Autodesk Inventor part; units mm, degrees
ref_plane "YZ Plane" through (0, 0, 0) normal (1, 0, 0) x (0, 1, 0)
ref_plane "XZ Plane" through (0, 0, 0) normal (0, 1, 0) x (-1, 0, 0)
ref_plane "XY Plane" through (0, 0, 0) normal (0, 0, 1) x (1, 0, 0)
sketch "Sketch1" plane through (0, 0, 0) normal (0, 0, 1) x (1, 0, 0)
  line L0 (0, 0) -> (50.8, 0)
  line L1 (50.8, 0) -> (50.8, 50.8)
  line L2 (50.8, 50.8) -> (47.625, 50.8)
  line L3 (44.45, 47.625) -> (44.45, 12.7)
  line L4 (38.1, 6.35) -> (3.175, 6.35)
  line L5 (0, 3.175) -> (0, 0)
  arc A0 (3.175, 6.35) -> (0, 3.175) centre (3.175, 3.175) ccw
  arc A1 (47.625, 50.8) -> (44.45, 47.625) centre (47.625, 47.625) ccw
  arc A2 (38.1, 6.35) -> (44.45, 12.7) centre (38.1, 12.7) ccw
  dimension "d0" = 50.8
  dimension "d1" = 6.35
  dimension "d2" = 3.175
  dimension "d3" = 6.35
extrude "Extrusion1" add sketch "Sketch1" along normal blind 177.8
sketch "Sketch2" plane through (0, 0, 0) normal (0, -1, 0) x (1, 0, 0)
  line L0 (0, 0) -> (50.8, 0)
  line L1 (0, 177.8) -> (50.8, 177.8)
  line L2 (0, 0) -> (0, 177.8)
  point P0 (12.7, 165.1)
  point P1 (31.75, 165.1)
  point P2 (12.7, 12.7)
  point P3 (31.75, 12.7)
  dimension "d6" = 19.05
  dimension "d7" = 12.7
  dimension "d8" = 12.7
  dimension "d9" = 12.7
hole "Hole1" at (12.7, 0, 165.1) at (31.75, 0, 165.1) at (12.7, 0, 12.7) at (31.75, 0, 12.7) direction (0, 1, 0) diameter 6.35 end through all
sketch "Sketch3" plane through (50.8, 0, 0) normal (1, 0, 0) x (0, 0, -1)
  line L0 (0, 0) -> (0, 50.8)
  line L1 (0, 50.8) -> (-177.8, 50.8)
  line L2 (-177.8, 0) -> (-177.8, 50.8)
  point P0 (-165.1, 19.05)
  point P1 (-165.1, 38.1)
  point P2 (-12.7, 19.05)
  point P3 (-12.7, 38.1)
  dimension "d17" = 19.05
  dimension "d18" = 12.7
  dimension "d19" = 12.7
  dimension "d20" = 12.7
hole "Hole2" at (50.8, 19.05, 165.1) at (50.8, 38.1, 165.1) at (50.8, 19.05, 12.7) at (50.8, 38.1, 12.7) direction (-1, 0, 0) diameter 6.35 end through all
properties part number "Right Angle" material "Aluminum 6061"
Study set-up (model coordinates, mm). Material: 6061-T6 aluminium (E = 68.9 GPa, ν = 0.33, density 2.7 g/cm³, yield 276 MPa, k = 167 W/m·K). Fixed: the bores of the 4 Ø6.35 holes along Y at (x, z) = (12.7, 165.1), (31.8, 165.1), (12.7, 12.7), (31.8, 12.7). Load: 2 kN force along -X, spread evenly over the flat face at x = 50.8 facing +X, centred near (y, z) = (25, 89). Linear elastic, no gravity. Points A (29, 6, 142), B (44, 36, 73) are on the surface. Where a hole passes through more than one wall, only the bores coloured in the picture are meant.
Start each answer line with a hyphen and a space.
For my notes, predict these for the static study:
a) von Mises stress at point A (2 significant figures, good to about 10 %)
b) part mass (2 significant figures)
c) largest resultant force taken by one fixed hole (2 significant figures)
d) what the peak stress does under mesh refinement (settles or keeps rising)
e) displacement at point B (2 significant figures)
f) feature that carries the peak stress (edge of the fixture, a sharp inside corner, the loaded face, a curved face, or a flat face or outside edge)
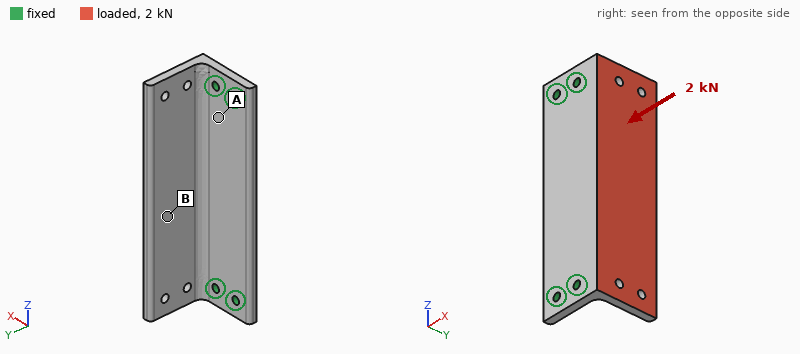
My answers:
- 30 MPa
- 290 g
- 1.0 kN
- keeps rising
- 0.18 mm
- edge of the fixture
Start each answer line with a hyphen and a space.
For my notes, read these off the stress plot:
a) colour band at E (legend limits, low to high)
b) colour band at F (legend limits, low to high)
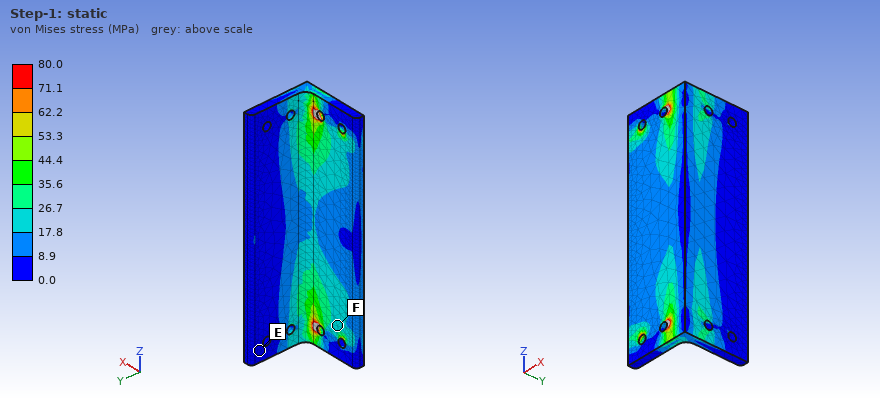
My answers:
- 0.0 to 8.9 MPa
- 17.8 to 26.7 MPa
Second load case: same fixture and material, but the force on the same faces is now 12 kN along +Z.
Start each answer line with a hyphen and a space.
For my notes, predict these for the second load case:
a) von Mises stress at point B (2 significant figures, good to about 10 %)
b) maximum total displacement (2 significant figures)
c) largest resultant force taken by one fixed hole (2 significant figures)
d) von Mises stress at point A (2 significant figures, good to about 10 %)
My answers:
- 11 MPa
- 66 µm
- 4.9 kN
- 25 MPa
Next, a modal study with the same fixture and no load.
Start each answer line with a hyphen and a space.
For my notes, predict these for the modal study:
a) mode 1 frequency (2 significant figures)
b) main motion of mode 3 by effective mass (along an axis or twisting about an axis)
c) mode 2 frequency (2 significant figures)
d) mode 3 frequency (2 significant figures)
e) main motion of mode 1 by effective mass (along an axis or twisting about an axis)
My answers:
- 1300 Hz
- along Y
- 2100 Hz
- 2500 Hz
- along X
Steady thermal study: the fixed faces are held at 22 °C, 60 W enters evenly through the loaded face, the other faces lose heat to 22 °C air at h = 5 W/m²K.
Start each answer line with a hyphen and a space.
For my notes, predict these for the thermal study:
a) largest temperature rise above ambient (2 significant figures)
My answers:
- 21 K
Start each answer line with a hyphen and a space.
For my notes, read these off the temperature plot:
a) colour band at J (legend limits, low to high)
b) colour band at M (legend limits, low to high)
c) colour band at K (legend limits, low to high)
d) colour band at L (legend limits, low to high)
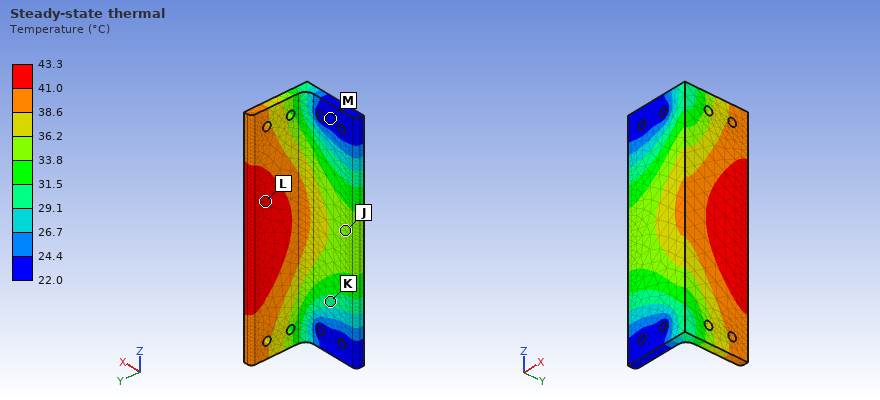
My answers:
- 33.8 to 36.2 °C
- 22.0 to 24.4 °C
- 29.1 to 31.5 °C
- 41.0 to 43.3 °C
